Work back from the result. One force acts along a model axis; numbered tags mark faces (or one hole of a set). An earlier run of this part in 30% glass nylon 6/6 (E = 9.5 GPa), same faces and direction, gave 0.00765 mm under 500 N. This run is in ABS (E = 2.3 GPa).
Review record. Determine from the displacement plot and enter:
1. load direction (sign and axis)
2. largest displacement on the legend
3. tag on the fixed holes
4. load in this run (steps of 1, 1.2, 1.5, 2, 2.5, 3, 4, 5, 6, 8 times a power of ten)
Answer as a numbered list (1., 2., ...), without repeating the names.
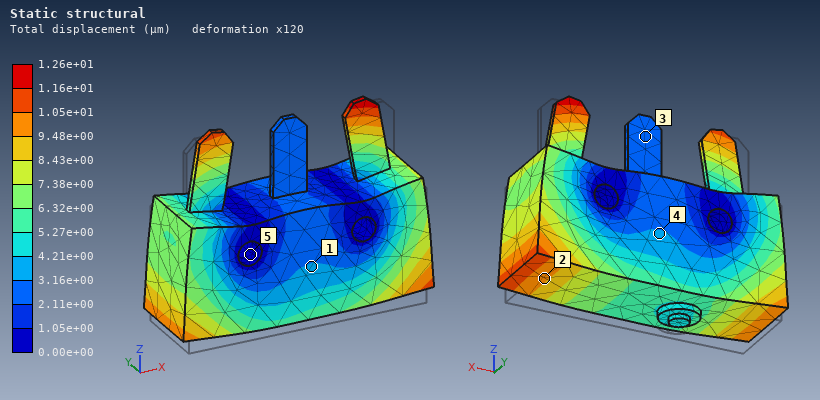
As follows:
1. +Z
2. 1.26e+01 µm
3. 5
4. 200 N
